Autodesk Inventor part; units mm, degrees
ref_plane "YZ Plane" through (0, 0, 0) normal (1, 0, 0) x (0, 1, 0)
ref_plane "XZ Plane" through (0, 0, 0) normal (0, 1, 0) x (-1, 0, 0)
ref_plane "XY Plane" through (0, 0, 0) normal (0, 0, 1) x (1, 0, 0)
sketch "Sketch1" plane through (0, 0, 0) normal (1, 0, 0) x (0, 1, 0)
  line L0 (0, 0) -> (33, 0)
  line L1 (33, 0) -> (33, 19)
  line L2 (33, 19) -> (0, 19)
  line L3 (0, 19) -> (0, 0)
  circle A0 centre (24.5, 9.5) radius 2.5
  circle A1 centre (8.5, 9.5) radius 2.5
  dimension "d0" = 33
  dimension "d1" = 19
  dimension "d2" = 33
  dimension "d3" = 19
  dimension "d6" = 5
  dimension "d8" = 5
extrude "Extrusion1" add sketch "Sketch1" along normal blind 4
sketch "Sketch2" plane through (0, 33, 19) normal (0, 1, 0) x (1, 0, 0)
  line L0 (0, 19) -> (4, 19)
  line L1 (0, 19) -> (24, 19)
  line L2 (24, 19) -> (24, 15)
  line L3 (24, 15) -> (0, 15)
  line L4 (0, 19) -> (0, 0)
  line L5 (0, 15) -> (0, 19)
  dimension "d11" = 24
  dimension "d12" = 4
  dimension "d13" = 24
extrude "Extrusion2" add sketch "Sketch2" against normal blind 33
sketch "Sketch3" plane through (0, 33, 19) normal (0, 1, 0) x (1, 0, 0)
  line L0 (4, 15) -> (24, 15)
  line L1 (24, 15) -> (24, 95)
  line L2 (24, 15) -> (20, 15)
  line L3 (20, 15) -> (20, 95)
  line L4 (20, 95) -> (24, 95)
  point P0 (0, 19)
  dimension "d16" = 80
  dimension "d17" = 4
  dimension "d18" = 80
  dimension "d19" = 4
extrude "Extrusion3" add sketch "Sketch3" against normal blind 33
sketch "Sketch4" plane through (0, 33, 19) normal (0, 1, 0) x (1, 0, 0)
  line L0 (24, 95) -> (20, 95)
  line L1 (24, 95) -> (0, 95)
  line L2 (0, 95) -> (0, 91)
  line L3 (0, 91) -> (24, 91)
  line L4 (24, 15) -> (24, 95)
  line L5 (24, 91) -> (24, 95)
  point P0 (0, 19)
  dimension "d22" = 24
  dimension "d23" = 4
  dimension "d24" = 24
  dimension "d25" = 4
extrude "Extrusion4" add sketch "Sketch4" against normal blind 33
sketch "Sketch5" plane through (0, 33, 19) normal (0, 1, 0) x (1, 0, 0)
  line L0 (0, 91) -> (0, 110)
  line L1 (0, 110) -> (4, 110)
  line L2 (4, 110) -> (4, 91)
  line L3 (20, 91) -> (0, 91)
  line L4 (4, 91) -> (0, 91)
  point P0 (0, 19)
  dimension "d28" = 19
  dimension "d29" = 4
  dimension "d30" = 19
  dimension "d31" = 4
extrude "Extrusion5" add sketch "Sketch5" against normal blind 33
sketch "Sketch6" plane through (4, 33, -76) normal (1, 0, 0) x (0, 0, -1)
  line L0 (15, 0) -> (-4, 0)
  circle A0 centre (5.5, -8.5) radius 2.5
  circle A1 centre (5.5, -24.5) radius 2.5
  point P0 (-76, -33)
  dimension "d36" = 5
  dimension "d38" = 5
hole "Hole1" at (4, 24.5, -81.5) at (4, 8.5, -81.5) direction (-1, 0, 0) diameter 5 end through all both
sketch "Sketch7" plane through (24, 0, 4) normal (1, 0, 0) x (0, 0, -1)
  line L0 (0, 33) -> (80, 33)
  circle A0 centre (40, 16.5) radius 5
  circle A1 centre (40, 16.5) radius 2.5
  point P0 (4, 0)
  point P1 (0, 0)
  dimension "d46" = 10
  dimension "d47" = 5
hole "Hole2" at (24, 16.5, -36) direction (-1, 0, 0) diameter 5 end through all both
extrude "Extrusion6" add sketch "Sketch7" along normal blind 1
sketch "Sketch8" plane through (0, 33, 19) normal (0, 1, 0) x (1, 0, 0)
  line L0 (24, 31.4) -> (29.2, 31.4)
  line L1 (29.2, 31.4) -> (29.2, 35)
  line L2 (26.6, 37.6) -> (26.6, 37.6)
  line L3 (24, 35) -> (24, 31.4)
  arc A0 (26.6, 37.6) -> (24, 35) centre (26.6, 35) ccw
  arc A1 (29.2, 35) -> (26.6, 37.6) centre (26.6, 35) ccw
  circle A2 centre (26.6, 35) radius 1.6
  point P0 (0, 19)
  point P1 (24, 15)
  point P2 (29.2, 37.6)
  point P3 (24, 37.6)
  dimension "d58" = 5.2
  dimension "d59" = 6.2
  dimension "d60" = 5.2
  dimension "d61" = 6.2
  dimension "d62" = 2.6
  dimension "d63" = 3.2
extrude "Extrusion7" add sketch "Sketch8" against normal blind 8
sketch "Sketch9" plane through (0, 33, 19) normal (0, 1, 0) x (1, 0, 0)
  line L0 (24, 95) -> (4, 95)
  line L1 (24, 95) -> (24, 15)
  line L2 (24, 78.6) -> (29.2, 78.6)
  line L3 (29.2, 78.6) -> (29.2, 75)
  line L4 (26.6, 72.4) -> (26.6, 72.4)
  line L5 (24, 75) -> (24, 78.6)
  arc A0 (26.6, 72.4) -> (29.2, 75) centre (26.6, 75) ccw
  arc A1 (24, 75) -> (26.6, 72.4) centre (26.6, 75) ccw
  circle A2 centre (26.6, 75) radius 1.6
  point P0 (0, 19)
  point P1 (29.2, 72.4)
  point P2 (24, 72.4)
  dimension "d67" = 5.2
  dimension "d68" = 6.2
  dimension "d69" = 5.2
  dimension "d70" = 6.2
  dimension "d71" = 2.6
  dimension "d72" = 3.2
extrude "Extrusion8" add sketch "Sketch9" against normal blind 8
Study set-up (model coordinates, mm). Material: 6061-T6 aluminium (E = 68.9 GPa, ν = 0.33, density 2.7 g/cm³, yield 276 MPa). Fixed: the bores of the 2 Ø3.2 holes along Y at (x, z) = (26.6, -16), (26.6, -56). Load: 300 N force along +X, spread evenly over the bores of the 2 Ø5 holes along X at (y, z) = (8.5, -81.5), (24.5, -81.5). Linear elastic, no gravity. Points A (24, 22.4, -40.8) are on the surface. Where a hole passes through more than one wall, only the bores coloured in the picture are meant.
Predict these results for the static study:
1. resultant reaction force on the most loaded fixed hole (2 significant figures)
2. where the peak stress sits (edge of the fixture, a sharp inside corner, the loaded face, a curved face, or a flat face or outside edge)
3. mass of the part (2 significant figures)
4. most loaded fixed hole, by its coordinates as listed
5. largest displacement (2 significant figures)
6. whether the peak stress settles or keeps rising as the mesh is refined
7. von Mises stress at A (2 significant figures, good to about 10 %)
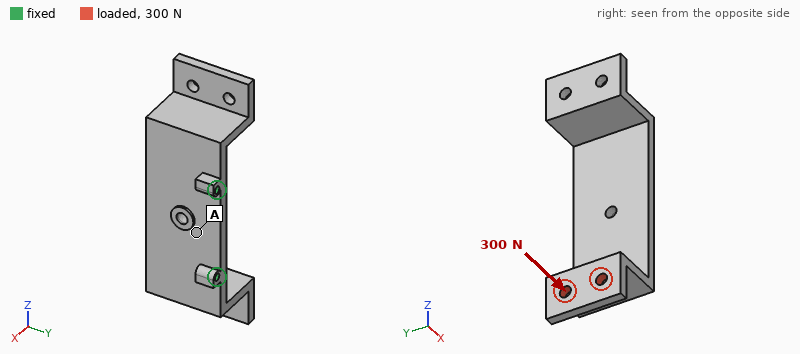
580 N
a sharp inside corner
53 g
(26.6, -56)
0.53 mm
keeps rising
17 MPa
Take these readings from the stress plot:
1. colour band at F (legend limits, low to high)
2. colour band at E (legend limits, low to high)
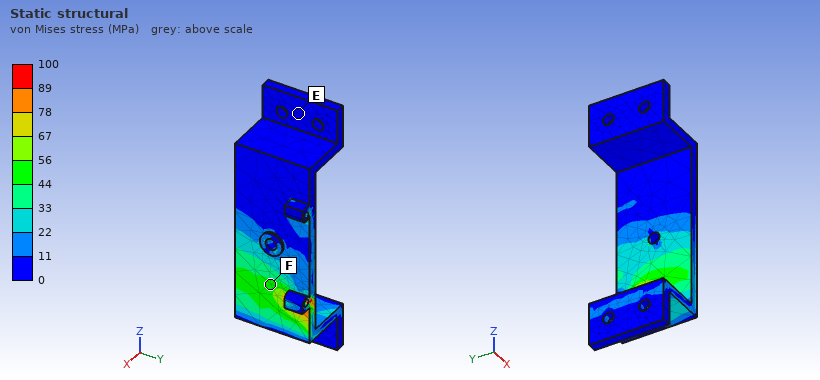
44 to 56 MPa
0 to 11 MPa
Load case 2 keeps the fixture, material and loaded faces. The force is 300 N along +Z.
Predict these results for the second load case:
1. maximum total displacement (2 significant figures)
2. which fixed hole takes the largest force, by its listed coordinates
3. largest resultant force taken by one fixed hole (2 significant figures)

0.49 mm
(26.6, -16)
480 N
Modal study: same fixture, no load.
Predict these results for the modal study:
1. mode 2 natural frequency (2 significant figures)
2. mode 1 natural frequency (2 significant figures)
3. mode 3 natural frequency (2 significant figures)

1300 Hz
1300 Hz
1700 Hz
